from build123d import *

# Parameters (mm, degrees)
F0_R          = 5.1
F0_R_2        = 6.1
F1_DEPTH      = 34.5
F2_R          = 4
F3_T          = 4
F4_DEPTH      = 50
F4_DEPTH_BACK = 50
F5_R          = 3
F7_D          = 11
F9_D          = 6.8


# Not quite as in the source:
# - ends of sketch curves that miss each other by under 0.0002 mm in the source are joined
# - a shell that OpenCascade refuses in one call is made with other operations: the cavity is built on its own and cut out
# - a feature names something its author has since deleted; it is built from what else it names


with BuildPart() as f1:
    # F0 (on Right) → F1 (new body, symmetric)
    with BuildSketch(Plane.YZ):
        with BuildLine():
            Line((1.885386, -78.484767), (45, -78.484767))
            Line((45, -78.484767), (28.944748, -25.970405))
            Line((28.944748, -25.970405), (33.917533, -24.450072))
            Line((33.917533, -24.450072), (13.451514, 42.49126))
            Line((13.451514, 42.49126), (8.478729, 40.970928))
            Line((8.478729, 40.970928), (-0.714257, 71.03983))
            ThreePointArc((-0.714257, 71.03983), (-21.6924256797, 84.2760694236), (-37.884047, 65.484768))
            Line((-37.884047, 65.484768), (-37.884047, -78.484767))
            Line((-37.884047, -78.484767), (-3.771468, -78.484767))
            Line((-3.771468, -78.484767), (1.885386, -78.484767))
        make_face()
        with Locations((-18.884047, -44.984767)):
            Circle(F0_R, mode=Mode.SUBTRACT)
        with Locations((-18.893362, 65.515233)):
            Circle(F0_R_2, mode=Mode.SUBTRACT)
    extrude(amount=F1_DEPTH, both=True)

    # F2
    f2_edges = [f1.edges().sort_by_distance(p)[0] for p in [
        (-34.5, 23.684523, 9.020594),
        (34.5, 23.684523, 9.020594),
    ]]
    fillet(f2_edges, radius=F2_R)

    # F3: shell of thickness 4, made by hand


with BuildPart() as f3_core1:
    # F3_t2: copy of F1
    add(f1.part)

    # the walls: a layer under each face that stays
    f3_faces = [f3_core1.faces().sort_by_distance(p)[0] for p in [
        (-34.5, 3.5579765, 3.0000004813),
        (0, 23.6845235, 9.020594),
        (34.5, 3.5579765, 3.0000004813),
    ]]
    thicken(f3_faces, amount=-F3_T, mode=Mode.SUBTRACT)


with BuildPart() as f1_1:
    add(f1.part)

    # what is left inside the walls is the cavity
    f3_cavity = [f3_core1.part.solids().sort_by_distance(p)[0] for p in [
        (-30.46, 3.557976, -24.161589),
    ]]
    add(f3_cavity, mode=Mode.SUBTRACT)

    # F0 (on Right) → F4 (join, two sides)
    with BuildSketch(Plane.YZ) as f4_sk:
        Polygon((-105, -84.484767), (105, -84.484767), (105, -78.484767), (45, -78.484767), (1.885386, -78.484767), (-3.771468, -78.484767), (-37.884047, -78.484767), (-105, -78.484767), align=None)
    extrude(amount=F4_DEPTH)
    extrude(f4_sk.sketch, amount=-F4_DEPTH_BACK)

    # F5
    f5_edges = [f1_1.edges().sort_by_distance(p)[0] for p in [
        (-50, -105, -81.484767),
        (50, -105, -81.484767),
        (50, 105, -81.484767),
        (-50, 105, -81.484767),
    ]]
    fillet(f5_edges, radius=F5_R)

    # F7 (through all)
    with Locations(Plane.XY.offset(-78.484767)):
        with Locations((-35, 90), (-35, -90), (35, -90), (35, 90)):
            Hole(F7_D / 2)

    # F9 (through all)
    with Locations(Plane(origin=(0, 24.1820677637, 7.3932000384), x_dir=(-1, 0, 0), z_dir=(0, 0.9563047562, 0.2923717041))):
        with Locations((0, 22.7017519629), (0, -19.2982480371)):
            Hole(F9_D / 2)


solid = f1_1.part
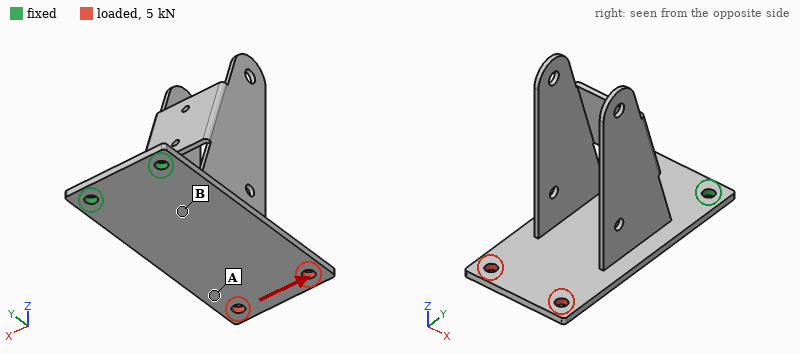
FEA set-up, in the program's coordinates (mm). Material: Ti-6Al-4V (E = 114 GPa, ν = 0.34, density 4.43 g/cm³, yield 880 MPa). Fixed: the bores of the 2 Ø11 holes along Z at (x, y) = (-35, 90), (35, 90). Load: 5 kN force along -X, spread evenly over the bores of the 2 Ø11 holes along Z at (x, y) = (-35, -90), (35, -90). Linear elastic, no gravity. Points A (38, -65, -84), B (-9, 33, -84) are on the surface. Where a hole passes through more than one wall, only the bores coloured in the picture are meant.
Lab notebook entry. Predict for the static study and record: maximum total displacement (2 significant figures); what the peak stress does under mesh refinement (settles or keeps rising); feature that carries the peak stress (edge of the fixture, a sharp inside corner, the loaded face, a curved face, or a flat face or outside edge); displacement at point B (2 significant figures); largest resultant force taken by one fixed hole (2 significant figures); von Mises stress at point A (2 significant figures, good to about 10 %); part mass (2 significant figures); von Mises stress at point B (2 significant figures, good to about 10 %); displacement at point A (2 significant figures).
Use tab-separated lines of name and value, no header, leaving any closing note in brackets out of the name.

maximum total displacement	0.24 mm
what the peak stress does under mesh refinement	keeps rising
feature that carries the peak stress	edge of the fixture
displacement at point B	0.038 mm
largest resultant force taken by one fixed hole	12 kN
von Mises stress at point A	11 MPa
part mass	960 g
von Mises stress at point B	28 MPa
displacement at point A	0.18 mm
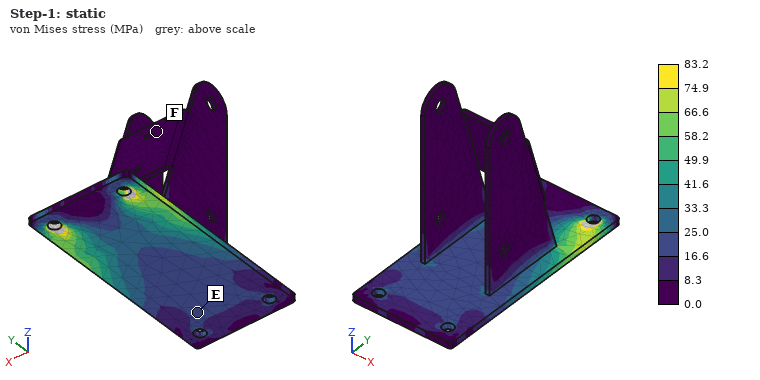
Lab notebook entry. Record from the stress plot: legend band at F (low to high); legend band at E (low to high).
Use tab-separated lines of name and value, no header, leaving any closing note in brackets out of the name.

legend band at F	0.0 to 8.3 MPa
legend band at E	16.6 to 25.0 MPa
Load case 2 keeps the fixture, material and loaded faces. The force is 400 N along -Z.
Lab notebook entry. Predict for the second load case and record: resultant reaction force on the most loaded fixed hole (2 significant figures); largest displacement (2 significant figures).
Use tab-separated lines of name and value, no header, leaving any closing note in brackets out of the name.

resultant reaction force on the most loaded fixed hole	200 N
largest displacement	2.9 mm
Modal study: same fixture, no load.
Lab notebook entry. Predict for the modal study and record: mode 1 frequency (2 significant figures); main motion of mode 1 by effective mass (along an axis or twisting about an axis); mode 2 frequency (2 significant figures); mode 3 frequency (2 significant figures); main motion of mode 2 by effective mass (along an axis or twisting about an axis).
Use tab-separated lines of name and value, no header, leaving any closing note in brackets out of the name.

mode 1 frequency	100 Hz
main motion of mode 1 by effective mass	along Z
mode 2 frequency	270 Hz
mode 3 frequency	540 Hz
main motion of mode 2 by effective mass	along X
